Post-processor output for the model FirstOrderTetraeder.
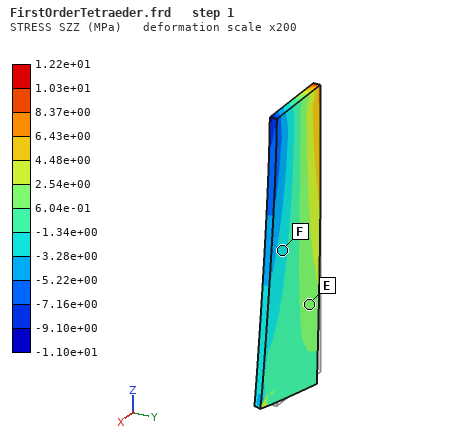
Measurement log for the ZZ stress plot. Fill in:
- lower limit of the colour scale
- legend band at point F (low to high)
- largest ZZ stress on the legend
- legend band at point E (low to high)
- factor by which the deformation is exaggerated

-1.10e+01 MPa
-3.28e+00 to -1.34e+00 MPa
1.22e+01 MPa
6.04e-01 to 2.54e+00 MPa
200
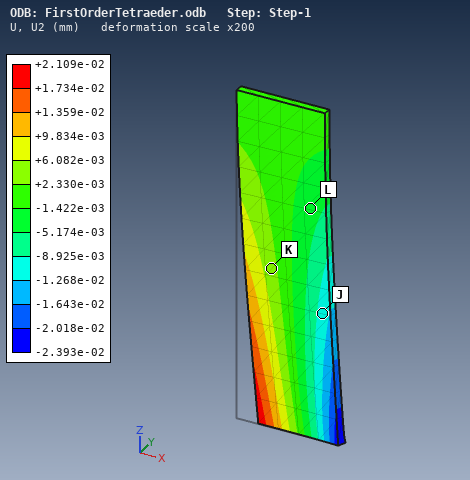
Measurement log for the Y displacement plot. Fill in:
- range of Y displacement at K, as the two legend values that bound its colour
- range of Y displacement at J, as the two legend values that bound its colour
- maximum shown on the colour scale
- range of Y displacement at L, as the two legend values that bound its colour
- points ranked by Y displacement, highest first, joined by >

+2.330e-03 to +6.082e-03 mm
-1.268e-02 to -8.925e-03 mm
+2.109e-02 mm
-5.174e-03 to -1.422e-03 mm
K > L > J
